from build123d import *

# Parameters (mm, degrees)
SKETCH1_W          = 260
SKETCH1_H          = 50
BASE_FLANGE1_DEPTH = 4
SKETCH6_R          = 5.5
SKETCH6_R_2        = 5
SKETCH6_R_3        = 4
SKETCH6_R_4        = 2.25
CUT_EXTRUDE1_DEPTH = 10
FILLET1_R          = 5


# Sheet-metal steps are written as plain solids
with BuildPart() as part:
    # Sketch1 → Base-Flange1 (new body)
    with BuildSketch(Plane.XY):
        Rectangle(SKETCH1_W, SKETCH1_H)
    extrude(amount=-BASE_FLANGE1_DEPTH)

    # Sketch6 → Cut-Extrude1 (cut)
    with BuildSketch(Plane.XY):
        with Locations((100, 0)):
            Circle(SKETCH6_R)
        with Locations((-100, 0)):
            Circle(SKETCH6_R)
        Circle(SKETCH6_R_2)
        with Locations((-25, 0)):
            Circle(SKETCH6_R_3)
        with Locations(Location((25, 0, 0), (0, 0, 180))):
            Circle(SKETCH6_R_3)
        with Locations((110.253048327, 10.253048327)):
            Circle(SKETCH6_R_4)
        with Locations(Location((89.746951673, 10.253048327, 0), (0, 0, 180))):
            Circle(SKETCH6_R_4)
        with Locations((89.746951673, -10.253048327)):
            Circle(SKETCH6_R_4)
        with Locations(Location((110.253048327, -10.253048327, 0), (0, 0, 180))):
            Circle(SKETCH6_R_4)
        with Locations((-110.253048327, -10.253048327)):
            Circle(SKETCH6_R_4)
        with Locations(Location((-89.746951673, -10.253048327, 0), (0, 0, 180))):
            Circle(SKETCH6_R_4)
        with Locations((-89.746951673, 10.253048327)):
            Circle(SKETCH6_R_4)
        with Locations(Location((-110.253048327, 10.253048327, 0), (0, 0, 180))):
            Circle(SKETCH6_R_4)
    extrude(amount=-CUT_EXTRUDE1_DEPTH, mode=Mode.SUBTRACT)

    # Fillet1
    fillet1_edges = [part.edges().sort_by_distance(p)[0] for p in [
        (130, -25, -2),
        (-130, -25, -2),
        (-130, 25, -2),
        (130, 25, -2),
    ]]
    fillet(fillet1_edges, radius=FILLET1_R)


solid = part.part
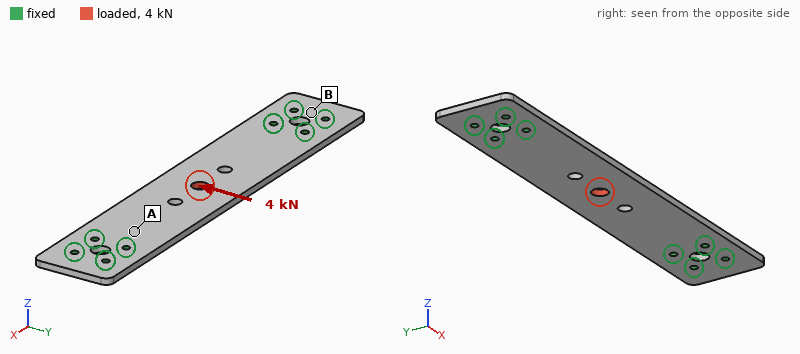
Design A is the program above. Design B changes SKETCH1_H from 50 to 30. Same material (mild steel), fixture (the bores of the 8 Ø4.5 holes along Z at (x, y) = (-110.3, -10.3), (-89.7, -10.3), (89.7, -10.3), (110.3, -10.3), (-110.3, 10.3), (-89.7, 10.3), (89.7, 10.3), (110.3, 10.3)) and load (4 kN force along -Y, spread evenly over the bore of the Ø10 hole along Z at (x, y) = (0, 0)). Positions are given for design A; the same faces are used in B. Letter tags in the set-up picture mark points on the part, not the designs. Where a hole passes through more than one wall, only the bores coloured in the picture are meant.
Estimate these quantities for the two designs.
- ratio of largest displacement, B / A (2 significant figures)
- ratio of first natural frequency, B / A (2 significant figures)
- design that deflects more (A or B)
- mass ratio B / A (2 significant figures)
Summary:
2.7
1.0
B
0.58
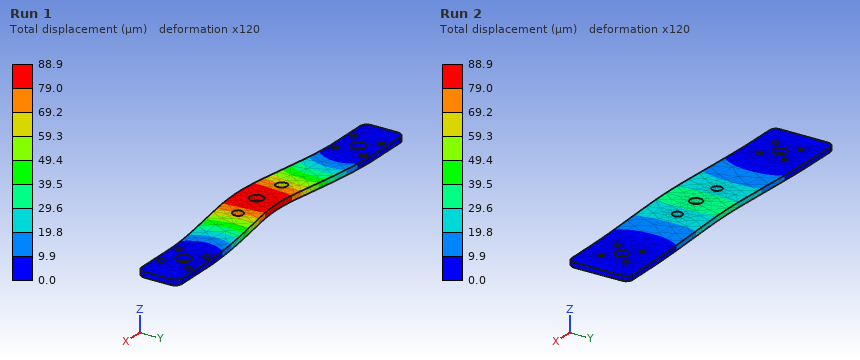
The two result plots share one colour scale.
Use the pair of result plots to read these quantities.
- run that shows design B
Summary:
Run 1
